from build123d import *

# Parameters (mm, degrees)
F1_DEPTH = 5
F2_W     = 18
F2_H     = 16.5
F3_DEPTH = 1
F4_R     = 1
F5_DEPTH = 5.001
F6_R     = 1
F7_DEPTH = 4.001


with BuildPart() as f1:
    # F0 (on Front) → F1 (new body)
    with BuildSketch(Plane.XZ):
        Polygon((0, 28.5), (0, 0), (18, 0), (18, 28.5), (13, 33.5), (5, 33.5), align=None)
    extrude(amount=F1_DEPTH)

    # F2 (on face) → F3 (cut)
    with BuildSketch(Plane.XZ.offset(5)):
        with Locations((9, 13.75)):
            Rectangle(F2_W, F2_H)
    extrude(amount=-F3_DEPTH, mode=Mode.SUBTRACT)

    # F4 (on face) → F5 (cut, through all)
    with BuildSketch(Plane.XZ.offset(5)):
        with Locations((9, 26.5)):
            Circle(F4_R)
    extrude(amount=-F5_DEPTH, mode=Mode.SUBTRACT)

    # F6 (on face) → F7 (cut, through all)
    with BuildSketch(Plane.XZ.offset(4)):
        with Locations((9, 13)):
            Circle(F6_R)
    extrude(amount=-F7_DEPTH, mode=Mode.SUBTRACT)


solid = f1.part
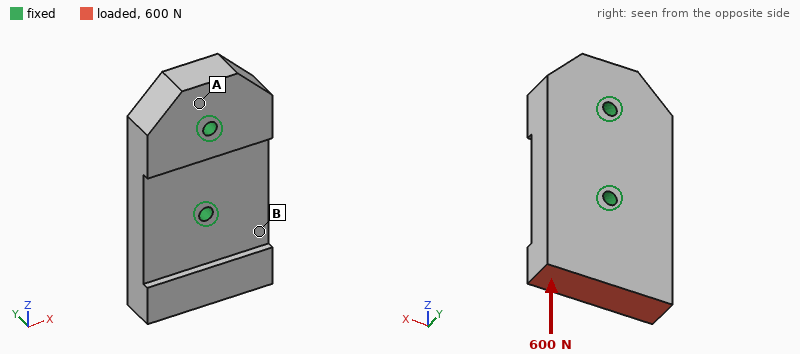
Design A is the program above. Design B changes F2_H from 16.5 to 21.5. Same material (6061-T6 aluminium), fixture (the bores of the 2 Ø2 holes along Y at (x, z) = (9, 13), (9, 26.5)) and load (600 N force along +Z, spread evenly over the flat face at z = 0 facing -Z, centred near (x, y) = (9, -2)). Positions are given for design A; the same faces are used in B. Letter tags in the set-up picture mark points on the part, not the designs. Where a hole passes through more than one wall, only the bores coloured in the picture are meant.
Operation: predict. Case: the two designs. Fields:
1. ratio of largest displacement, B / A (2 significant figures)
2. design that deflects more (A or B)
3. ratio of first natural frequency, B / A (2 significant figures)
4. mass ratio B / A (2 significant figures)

1.1
B
1.0
0.96
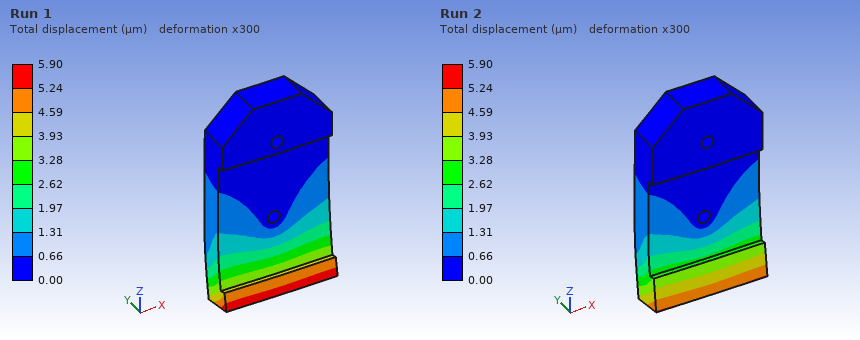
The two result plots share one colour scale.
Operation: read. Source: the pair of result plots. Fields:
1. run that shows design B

Run 1
